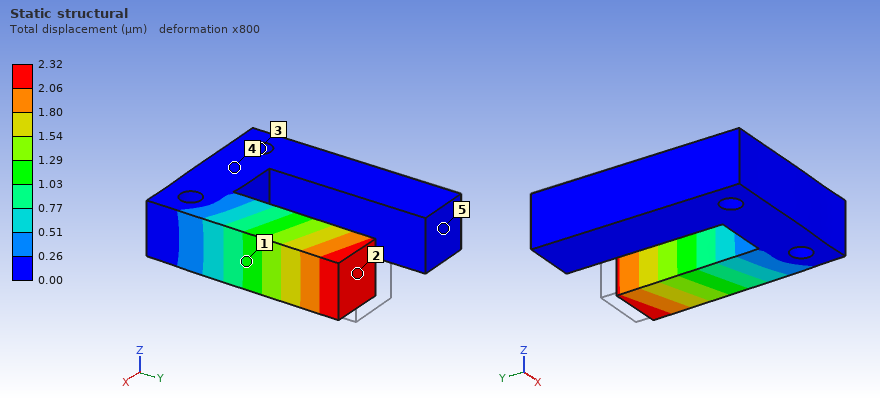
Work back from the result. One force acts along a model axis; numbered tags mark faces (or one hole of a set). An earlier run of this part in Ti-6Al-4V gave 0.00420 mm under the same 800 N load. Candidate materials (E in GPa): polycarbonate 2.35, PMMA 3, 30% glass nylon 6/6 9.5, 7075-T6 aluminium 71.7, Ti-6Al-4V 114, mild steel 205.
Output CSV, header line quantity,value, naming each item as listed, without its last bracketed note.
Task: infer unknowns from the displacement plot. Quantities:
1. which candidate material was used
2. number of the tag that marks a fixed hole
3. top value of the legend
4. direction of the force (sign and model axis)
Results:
quantity,value
which candidate material was used,mild steel
number of the tag that marks a fixed hole,3
top value of the legend,2.32 µm
direction of the force,-Y
